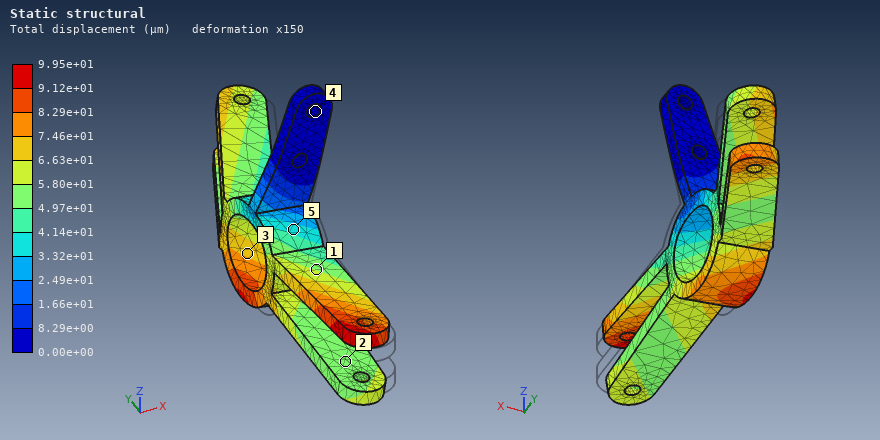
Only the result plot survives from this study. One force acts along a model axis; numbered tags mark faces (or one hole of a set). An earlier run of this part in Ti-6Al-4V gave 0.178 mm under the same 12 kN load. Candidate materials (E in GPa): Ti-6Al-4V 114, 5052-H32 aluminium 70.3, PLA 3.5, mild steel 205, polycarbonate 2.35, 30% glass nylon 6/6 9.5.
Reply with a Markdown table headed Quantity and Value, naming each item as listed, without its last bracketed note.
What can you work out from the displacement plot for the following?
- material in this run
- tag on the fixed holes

| Quantity | Value |
|---|---|
| material in this run | mild steel |
| tag on the fixed holes | 4 |
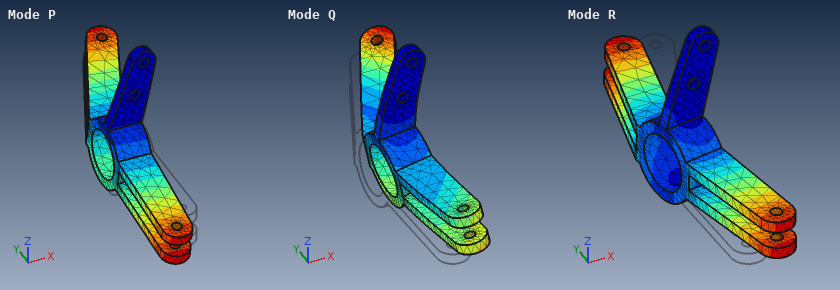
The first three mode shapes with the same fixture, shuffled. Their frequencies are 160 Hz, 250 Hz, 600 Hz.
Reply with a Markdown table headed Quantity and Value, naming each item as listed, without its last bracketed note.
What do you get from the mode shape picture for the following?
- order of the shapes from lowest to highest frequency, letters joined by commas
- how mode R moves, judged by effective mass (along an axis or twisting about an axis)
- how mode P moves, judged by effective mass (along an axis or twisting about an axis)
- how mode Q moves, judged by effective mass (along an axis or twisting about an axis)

| Quantity | Value |
|---|---|
| order of the shapes from lowest to highest frequency, letters joined by commas | P, R, Q |
| how mode R moves, judged by effective mass | twisting about Z |
| how mode P moves, judged by effective mass | along Y |
| how mode Q moves, judged by effective mass | along X |
